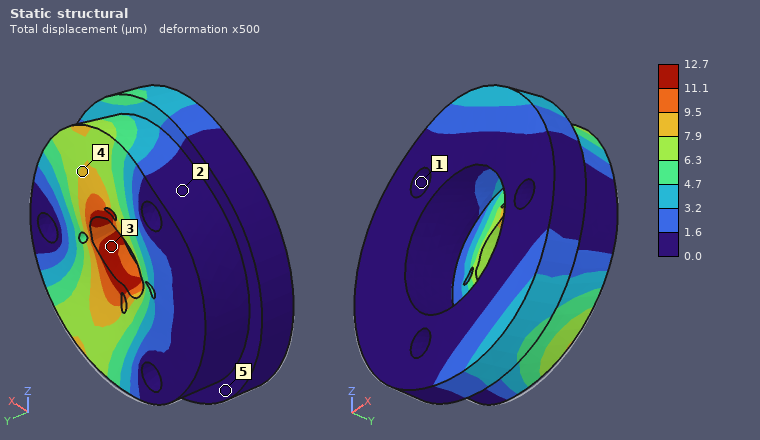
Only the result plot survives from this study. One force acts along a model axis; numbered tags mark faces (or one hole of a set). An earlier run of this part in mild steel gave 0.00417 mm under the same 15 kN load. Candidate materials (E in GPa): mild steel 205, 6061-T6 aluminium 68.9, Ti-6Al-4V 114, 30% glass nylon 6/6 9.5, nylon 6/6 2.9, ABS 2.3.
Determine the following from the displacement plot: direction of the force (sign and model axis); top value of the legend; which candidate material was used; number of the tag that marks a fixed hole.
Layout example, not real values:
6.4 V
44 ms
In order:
+Z
12.7 µm
6061-T6 aluminium
1
